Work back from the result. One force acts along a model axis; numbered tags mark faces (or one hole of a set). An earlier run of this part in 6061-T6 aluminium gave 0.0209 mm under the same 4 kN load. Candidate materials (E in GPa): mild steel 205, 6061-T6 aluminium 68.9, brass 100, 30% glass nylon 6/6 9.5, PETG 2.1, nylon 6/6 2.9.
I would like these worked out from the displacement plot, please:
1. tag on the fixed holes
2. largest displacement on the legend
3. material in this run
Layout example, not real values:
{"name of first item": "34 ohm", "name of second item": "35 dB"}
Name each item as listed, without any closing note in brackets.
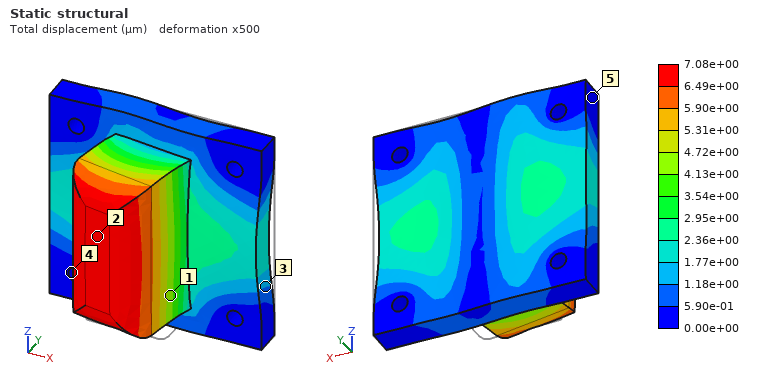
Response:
{"tag on the fixed holes": "4", "largest displacement on the legend": "7.08e+00 µm", "material in this run": "mild steel"}
